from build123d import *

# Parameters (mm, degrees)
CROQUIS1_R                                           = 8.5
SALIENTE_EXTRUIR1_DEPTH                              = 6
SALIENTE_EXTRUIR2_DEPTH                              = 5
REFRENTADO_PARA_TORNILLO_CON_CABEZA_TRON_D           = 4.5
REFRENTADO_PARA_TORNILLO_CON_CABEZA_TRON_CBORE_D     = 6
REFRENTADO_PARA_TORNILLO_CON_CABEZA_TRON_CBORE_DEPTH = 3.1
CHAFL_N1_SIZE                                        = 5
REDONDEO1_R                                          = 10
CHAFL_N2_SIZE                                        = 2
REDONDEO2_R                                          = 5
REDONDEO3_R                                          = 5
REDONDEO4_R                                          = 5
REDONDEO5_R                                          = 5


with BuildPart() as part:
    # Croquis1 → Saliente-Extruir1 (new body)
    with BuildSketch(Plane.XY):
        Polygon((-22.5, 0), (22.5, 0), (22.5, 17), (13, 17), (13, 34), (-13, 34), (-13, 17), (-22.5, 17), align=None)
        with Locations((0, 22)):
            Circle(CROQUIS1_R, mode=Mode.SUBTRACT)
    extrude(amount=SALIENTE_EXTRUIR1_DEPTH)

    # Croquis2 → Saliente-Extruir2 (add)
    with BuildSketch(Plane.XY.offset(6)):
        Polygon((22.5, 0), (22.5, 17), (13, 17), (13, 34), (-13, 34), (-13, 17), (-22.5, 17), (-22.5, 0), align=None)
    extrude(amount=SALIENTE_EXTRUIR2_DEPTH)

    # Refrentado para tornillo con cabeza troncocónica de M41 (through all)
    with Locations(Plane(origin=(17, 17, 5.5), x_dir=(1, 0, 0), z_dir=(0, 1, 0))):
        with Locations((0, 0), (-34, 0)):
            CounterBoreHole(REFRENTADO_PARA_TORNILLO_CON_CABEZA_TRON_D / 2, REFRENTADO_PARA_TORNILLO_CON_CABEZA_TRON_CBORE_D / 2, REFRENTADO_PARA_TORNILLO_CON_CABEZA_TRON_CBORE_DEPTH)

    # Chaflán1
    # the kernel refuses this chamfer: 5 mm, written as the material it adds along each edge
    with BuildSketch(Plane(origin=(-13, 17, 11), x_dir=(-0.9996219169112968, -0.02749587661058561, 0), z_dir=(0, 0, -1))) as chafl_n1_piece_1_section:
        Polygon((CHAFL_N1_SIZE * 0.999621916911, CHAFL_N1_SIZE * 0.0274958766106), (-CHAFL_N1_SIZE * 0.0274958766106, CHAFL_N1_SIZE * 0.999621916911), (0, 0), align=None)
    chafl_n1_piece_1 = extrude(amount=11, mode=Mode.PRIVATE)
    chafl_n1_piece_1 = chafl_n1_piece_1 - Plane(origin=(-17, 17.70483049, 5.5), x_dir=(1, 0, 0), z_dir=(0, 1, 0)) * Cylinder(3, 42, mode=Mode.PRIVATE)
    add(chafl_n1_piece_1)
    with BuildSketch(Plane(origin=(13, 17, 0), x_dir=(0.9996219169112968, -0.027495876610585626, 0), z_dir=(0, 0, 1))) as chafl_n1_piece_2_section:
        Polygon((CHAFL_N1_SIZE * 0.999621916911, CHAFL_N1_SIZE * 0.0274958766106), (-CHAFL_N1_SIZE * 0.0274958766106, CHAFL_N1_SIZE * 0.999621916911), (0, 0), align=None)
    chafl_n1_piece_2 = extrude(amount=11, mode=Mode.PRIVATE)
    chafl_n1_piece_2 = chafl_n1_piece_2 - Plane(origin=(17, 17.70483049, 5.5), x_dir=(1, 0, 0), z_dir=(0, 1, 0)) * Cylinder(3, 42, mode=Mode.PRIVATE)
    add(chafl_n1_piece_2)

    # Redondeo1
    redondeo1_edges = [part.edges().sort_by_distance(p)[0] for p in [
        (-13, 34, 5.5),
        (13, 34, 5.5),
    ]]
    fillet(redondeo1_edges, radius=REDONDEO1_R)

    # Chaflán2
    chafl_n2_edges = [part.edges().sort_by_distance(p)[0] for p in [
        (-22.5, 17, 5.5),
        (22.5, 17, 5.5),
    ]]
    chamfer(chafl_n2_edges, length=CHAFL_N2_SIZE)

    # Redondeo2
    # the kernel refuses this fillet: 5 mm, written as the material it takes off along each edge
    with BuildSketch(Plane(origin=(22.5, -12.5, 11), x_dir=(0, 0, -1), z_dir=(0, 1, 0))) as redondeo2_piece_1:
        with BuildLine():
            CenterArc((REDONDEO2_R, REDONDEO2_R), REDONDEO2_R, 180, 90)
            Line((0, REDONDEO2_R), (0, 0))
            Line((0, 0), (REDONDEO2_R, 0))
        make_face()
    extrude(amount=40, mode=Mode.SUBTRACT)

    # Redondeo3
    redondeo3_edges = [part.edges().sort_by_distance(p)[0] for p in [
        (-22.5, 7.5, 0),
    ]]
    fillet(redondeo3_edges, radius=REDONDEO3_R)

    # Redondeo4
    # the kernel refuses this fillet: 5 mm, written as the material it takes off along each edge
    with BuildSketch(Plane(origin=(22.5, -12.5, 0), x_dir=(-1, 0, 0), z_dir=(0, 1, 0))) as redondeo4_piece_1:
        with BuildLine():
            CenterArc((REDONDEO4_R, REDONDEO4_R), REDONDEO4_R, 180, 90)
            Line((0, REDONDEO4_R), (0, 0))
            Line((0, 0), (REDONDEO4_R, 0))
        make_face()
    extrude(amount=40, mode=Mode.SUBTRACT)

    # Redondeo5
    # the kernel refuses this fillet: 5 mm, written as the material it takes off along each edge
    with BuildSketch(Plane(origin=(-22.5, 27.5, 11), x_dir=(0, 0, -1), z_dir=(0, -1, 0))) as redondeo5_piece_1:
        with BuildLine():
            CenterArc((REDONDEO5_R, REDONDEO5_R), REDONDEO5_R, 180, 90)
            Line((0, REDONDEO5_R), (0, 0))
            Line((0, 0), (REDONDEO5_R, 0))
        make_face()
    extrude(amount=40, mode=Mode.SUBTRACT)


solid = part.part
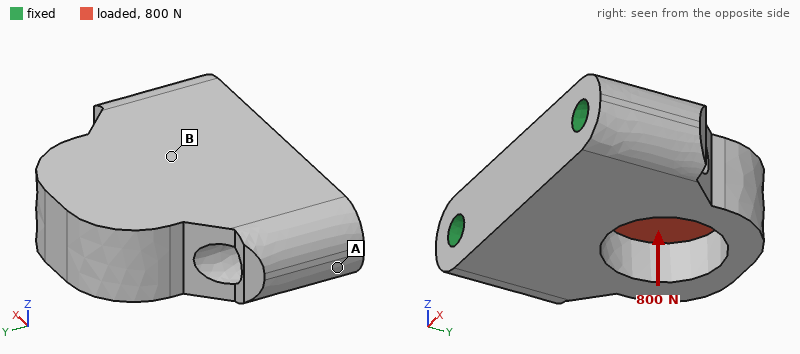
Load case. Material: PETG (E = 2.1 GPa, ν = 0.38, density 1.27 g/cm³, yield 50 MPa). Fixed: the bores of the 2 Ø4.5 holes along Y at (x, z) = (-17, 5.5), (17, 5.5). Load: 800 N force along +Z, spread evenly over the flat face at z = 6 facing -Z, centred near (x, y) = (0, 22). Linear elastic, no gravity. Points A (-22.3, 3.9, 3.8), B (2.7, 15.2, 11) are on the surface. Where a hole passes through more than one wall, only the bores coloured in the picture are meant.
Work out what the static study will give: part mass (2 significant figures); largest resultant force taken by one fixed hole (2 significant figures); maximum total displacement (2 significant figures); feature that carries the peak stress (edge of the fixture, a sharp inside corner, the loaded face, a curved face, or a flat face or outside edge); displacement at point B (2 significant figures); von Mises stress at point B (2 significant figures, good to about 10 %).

14 g
400 N
0.61 mm
edge of the fixture
0.20 mm
10 MPa
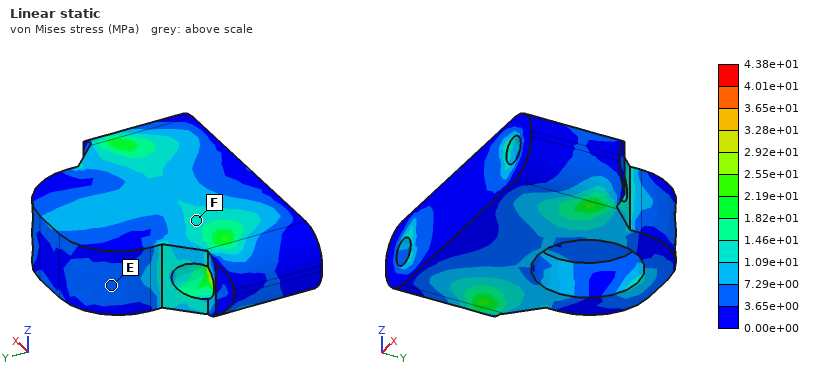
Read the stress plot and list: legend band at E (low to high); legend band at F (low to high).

3.65e+00 to 7.29e+00 MPa
1.09e+01 to 1.46e+01 MPa
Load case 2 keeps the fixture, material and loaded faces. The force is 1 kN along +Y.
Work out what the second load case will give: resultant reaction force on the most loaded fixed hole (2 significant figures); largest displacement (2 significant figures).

540 N
81 µm
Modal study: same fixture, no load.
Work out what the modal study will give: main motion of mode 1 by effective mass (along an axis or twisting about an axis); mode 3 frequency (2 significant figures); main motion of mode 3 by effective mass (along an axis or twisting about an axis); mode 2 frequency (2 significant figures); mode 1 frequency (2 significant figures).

along Z
7700 Hz
along Z
5800 Hz
2900 Hz
